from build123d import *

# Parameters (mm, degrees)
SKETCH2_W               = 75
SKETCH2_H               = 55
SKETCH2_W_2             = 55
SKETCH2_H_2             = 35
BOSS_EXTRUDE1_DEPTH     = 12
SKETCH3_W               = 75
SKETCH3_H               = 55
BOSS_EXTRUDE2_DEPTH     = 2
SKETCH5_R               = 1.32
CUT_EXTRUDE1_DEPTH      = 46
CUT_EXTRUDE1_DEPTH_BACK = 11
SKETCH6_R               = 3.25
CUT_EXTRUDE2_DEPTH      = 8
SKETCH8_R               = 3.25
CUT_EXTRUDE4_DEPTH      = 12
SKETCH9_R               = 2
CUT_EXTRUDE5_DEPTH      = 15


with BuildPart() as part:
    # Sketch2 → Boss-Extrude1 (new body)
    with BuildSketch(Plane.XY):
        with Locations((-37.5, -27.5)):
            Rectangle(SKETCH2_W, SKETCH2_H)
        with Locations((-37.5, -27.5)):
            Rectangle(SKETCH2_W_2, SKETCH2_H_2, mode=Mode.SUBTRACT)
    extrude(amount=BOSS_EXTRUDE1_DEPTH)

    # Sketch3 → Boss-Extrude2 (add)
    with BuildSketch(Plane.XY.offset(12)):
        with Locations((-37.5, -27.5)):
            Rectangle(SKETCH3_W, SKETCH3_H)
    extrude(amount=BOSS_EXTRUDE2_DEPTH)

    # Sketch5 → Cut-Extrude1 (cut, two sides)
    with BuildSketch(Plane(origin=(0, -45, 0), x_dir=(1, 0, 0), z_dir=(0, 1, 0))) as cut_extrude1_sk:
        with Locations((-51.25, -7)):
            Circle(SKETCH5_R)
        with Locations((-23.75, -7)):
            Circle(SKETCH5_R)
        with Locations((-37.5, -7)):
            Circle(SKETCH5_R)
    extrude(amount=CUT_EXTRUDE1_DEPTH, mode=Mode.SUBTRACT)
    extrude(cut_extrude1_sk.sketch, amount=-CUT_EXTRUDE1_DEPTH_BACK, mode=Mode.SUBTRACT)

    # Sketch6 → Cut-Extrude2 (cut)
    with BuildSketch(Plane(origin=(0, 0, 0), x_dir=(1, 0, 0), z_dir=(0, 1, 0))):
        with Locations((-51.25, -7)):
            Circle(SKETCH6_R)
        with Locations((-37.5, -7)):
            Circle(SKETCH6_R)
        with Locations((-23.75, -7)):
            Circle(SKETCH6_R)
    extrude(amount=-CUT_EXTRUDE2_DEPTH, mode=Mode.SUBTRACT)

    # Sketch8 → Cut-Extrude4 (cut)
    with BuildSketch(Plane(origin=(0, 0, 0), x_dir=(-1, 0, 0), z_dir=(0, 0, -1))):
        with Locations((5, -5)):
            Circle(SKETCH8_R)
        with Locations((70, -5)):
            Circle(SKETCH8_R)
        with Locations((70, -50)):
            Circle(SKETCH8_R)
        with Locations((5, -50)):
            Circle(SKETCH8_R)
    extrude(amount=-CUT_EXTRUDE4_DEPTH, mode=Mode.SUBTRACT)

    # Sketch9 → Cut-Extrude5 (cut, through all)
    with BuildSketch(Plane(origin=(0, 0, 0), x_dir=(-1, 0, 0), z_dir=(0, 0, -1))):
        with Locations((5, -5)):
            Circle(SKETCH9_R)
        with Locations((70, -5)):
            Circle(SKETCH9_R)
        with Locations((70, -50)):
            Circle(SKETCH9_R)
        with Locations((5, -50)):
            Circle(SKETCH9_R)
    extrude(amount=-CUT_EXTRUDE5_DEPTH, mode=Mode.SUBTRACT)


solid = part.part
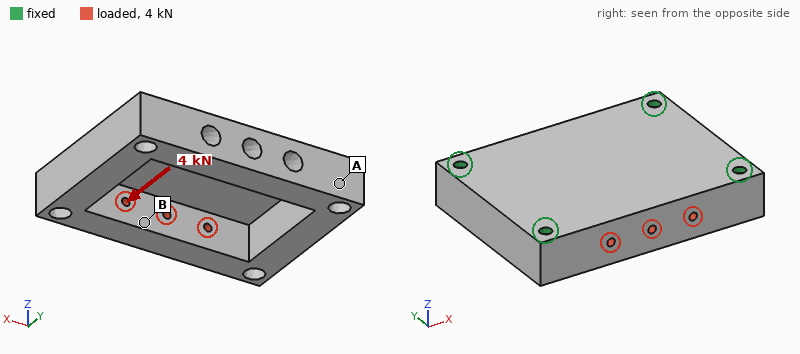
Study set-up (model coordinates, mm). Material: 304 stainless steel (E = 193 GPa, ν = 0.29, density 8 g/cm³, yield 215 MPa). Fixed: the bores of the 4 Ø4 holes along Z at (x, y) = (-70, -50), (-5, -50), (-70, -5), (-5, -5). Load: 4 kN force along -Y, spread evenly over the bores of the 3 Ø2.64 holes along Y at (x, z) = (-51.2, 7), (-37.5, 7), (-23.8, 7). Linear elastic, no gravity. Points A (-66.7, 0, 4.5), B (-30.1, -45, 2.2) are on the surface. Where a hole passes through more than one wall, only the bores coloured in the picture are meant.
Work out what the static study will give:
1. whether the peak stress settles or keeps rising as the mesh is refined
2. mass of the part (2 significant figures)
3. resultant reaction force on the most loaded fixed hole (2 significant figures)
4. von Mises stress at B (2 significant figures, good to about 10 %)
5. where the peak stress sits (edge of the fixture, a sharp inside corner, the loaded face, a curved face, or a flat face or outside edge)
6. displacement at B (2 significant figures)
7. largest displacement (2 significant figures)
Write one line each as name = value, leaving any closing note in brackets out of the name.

whether the peak stress settles or keeps rising as the mesh is refined = keeps rising
mass of the part = 260 g
resultant reaction force on the most loaded fixed hole = 1.3 kN
von Mises stress at B = 29 MPa
where the peak stress sits = edge of the fixture
displacement at B = 17 µm
largest displacement = 21 µm
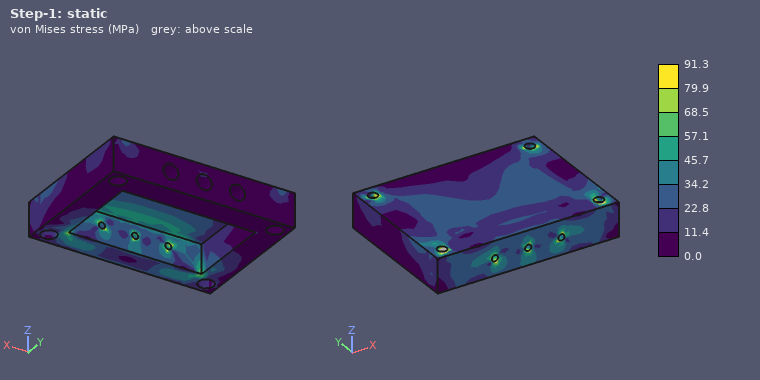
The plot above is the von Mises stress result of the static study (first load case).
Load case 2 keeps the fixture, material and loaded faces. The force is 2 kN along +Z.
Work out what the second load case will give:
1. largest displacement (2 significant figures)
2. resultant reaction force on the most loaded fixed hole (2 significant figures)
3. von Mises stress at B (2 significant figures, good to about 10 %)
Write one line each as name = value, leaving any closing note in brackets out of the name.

largest displacement = 13 µm
resultant reaction force on the most loaded fixed hole = 1.5 kN
von Mises stress at B = 31 MPa
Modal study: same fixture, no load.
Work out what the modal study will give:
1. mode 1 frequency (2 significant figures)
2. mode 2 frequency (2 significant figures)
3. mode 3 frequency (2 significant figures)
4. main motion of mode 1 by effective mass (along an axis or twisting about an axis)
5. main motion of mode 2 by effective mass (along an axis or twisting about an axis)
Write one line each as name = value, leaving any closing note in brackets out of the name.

mode 1 frequency = 7200 Hz
mode 2 frequency = 9500 Hz
mode 3 frequency = 10 kHz
main motion of mode 1 by effective mass = along Z
main motion of mode 2 by effective mass = twisting about X
